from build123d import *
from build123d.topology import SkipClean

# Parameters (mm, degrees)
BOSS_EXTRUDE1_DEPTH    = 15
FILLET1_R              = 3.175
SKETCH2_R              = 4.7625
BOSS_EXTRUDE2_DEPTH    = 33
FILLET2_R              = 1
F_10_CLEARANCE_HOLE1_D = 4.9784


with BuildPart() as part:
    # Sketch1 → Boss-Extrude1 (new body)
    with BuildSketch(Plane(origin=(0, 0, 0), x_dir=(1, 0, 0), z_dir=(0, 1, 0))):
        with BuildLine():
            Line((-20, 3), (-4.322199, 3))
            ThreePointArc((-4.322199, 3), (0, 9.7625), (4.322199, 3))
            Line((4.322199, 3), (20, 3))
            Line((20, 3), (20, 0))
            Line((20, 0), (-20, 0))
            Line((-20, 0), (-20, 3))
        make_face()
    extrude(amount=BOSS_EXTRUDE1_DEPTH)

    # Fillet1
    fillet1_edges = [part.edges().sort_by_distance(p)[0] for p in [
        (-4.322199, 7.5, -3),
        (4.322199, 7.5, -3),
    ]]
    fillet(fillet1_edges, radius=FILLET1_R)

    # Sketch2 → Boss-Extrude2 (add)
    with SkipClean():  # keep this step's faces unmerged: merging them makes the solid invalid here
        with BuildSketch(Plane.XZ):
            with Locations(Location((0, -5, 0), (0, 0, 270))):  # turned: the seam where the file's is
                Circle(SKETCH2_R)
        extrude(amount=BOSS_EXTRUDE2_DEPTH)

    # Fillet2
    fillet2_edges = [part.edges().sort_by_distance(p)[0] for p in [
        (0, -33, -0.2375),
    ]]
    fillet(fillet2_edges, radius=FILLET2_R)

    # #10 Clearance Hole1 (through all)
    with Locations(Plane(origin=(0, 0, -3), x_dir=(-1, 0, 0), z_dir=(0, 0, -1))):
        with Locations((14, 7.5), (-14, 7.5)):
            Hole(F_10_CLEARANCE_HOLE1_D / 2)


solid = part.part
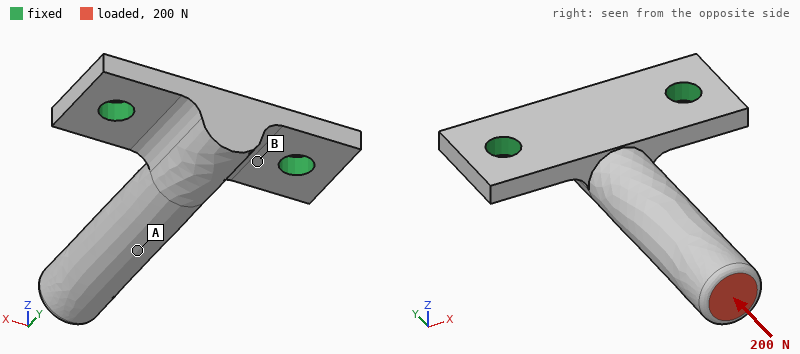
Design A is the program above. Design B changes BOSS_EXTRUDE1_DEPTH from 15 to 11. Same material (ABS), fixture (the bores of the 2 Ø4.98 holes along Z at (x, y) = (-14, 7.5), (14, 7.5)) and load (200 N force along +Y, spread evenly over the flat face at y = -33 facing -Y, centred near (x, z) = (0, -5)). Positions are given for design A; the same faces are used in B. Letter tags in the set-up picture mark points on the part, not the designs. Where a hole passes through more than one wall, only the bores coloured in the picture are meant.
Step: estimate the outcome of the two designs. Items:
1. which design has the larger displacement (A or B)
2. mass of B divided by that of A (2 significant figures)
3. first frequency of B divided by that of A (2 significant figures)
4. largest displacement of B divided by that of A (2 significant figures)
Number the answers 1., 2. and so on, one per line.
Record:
1. B
2. 0.85
3. 0.86
4. 1.5
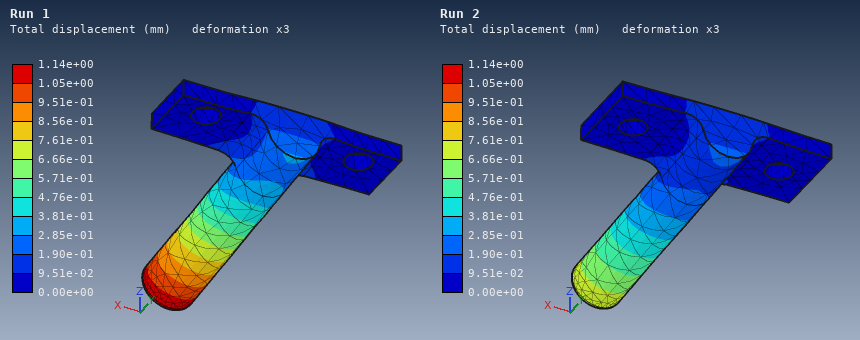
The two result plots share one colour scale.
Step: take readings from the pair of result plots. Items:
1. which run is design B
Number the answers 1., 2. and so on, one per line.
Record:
1. Run 1
